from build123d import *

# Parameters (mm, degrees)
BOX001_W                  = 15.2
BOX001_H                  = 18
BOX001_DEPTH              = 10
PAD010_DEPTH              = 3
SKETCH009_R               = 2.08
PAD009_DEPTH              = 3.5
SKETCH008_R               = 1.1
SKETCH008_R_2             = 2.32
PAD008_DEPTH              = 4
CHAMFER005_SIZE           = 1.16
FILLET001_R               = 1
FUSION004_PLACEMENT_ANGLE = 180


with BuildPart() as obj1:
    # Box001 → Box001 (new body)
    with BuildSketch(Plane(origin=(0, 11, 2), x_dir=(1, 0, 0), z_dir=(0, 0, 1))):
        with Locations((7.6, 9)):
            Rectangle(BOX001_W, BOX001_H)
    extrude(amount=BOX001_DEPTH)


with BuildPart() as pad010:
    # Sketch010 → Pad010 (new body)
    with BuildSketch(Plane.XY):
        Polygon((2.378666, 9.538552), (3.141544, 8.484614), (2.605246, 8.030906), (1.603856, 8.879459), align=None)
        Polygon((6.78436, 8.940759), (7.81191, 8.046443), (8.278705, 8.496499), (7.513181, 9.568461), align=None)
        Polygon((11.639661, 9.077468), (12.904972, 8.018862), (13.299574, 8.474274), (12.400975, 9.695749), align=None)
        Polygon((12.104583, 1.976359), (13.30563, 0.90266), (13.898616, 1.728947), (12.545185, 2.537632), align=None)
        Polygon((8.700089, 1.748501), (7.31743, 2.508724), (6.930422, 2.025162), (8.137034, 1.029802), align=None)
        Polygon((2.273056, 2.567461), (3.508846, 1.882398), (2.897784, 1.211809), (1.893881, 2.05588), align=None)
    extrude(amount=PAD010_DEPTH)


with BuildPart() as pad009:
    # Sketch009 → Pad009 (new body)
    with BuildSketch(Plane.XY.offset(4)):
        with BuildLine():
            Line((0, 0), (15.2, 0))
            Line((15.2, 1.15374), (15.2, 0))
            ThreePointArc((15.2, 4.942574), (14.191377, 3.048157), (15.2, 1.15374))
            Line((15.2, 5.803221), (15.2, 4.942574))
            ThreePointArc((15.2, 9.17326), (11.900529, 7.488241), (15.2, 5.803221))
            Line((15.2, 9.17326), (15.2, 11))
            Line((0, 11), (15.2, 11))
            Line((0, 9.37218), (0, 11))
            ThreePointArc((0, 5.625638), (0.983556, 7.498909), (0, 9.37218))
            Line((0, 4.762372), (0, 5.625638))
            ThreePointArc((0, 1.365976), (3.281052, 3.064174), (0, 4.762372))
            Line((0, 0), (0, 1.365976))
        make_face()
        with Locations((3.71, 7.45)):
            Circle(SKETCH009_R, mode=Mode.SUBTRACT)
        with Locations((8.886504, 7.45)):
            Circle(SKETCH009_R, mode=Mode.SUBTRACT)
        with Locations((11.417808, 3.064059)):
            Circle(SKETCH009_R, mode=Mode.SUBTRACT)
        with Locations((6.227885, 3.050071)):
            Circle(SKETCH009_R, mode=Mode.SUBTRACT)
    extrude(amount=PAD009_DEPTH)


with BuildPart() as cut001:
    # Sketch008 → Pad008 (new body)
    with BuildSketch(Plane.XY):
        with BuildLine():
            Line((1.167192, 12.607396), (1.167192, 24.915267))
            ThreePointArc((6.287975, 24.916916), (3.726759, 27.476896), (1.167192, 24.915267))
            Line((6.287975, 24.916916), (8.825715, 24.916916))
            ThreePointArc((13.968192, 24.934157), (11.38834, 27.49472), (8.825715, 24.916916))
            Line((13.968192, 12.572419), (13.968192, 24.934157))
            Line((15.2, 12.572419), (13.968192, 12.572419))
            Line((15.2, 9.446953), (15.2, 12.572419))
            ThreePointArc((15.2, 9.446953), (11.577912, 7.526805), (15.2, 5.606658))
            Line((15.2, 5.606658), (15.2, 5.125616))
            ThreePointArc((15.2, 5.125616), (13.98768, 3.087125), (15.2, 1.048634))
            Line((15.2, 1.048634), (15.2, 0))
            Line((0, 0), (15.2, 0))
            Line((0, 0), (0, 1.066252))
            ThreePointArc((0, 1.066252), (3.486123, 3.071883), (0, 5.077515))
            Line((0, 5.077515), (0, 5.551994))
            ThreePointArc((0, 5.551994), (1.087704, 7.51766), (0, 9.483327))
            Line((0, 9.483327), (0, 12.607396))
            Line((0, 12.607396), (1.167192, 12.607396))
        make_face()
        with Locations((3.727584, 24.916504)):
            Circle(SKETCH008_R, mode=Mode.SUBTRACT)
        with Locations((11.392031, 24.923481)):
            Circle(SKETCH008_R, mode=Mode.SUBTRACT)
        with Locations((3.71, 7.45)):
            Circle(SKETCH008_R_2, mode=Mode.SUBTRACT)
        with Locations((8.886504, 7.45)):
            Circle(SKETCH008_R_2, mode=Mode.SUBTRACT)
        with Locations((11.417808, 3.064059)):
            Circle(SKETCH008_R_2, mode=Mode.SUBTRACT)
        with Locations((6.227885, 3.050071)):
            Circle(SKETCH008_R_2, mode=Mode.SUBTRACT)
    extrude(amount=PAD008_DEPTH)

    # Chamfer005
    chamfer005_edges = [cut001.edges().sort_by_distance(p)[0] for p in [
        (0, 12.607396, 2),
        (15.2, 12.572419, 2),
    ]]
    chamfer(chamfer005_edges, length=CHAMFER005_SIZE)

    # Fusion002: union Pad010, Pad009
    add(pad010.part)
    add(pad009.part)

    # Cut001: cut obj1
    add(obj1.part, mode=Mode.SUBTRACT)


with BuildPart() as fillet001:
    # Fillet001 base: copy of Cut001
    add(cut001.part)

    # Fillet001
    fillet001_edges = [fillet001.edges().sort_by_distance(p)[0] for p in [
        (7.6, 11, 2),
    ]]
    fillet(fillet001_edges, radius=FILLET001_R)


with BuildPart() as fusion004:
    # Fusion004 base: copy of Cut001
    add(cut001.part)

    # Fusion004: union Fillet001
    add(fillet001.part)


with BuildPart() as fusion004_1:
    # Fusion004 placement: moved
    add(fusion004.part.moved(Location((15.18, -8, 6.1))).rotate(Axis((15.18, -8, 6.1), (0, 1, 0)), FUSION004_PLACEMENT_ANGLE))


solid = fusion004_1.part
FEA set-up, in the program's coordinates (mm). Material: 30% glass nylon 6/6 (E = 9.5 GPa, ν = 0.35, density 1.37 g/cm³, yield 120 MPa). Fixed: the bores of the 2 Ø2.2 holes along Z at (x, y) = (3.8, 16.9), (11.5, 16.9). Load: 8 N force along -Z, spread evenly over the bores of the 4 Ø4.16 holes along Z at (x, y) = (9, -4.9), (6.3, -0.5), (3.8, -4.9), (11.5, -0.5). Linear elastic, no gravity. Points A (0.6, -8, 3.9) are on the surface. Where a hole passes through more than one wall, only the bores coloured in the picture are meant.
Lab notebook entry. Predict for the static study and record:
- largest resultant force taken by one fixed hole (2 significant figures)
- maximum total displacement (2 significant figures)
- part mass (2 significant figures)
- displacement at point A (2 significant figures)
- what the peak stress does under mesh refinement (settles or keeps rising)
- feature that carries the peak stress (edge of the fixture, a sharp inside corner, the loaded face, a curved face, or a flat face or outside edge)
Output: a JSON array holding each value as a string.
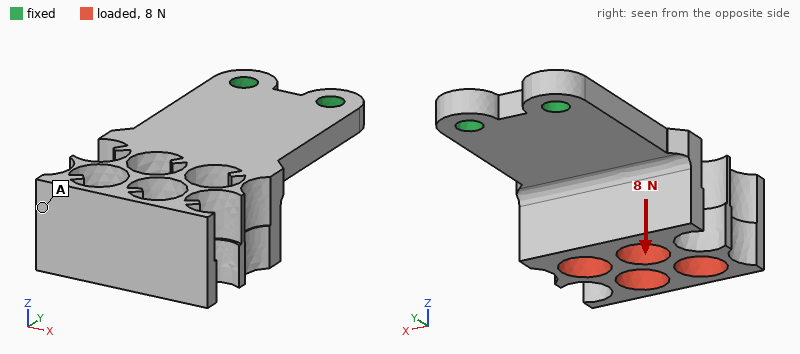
["4.0 N", "0.33 mm", "1.3 g", "0.31 mm", "keeps rising", "edge of the fixture"]
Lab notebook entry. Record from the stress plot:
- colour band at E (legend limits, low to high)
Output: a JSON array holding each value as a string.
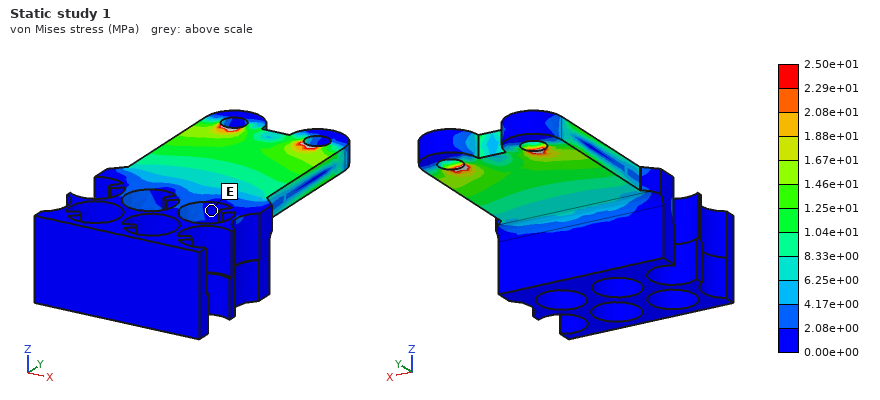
["0.00e+00 to 2.08e+00 MPa"]
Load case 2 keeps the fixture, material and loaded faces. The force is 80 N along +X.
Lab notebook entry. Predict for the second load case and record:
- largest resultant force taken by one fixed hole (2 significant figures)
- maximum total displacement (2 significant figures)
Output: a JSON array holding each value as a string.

["180 N", "0.38 mm"]
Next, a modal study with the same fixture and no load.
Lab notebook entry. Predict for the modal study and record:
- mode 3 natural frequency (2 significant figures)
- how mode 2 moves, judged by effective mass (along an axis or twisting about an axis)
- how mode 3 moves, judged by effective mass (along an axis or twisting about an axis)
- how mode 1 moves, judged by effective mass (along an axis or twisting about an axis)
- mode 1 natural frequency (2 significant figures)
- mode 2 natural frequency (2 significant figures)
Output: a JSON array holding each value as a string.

["5000 Hz", "along X", "along X", "along Z", "1000 Hz", "3200 Hz"]
